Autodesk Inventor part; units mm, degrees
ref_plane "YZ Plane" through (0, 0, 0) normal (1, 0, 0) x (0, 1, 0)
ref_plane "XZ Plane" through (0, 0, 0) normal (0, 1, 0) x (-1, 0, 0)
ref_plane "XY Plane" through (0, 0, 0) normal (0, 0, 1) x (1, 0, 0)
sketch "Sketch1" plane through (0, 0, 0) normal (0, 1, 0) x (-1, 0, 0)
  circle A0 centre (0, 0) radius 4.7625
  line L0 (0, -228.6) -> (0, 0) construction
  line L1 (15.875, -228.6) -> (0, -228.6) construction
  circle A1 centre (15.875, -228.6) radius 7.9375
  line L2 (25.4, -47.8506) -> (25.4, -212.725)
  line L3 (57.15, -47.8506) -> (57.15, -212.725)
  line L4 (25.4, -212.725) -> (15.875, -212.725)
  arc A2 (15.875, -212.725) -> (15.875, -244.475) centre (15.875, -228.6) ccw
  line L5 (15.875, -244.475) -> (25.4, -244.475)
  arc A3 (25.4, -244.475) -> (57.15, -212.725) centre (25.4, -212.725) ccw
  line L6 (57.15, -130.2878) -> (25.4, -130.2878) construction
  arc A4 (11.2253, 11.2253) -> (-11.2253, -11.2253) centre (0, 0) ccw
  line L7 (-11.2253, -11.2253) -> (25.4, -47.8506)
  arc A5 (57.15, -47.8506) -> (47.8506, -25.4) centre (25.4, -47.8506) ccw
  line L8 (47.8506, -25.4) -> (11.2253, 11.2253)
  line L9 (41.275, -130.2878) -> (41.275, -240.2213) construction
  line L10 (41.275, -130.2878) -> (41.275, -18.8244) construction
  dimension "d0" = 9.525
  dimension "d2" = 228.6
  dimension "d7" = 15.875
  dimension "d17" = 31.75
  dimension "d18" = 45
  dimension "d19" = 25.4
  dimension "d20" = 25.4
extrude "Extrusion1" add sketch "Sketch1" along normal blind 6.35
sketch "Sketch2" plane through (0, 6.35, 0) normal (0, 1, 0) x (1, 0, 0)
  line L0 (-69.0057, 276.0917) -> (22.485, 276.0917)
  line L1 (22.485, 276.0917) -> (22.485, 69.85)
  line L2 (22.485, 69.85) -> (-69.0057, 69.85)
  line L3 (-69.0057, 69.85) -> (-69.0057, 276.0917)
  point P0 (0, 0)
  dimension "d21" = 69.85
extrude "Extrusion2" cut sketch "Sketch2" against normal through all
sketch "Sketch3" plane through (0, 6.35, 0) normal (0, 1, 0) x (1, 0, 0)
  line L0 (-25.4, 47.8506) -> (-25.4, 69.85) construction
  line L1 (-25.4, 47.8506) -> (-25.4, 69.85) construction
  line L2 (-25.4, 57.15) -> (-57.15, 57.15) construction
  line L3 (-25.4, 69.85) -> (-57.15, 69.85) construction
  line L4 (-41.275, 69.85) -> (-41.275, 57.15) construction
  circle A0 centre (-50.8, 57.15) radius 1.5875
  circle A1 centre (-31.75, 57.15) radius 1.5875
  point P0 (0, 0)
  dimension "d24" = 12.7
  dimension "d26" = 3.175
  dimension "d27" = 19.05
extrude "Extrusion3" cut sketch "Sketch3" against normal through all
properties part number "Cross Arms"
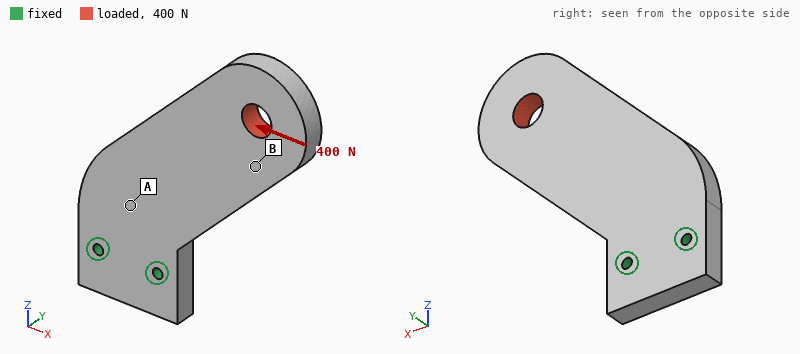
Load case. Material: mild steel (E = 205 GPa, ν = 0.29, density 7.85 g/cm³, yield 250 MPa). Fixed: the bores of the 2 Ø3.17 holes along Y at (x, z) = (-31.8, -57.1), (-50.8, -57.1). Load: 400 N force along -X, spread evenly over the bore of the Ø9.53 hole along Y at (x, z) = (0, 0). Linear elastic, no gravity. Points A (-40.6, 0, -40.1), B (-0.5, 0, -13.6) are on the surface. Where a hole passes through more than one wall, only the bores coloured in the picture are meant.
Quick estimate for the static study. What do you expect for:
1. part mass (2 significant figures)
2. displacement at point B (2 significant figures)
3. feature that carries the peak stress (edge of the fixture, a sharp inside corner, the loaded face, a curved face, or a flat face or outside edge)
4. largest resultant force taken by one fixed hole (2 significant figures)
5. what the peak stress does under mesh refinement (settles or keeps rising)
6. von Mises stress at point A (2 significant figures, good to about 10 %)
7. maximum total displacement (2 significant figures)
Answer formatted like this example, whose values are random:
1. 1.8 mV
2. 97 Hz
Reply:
1. 150 g
2. 11 µm
3. edge of the fixture
4. 1.1 kN
5. keeps rising
6. 8.4 MPa
7. 18 µm
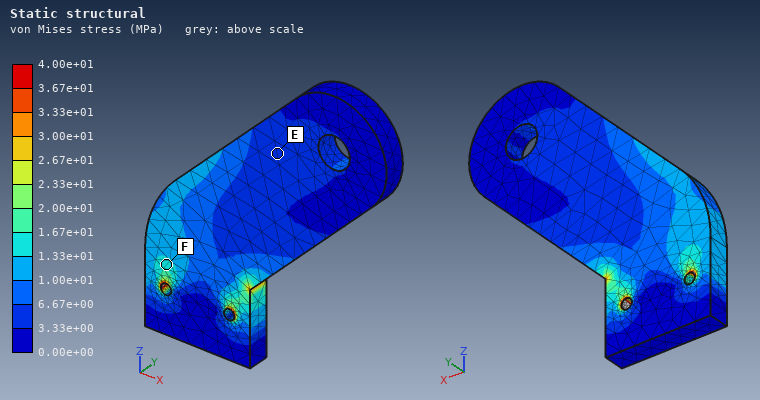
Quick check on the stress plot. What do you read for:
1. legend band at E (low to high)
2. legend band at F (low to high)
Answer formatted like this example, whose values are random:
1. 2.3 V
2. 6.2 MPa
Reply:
1. 3.33e+00 to 6.67e+00 MPa
2. 1.33e+01 to 1.67e+01 MPa
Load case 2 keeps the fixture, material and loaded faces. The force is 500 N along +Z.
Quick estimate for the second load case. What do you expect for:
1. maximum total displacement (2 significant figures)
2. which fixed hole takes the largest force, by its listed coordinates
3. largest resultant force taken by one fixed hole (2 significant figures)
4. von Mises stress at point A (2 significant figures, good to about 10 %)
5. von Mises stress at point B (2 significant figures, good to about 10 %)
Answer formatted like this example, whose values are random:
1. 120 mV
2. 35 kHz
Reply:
1. 19 µm
2. (-31.8, -57.1)
3. 1.3 kN
4. 5.8 MPa
5. 4.8 MPa
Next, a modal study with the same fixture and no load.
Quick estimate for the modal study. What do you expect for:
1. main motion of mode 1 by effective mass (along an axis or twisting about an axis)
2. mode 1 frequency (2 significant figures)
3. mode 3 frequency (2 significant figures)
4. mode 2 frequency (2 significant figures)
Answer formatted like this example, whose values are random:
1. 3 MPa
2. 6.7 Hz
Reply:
1. along Y
2. 790 Hz
3. 3400 Hz
4. 3300 Hz
